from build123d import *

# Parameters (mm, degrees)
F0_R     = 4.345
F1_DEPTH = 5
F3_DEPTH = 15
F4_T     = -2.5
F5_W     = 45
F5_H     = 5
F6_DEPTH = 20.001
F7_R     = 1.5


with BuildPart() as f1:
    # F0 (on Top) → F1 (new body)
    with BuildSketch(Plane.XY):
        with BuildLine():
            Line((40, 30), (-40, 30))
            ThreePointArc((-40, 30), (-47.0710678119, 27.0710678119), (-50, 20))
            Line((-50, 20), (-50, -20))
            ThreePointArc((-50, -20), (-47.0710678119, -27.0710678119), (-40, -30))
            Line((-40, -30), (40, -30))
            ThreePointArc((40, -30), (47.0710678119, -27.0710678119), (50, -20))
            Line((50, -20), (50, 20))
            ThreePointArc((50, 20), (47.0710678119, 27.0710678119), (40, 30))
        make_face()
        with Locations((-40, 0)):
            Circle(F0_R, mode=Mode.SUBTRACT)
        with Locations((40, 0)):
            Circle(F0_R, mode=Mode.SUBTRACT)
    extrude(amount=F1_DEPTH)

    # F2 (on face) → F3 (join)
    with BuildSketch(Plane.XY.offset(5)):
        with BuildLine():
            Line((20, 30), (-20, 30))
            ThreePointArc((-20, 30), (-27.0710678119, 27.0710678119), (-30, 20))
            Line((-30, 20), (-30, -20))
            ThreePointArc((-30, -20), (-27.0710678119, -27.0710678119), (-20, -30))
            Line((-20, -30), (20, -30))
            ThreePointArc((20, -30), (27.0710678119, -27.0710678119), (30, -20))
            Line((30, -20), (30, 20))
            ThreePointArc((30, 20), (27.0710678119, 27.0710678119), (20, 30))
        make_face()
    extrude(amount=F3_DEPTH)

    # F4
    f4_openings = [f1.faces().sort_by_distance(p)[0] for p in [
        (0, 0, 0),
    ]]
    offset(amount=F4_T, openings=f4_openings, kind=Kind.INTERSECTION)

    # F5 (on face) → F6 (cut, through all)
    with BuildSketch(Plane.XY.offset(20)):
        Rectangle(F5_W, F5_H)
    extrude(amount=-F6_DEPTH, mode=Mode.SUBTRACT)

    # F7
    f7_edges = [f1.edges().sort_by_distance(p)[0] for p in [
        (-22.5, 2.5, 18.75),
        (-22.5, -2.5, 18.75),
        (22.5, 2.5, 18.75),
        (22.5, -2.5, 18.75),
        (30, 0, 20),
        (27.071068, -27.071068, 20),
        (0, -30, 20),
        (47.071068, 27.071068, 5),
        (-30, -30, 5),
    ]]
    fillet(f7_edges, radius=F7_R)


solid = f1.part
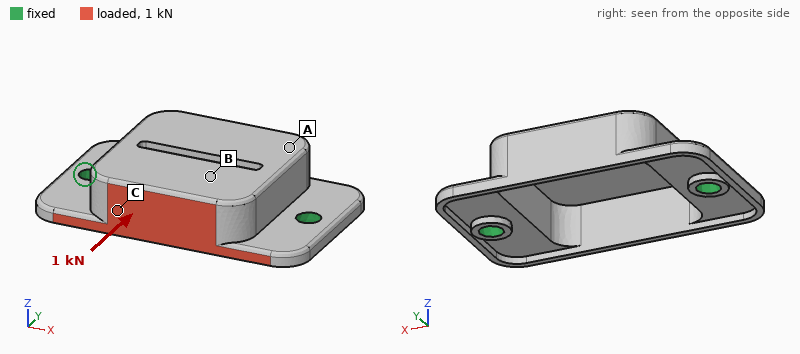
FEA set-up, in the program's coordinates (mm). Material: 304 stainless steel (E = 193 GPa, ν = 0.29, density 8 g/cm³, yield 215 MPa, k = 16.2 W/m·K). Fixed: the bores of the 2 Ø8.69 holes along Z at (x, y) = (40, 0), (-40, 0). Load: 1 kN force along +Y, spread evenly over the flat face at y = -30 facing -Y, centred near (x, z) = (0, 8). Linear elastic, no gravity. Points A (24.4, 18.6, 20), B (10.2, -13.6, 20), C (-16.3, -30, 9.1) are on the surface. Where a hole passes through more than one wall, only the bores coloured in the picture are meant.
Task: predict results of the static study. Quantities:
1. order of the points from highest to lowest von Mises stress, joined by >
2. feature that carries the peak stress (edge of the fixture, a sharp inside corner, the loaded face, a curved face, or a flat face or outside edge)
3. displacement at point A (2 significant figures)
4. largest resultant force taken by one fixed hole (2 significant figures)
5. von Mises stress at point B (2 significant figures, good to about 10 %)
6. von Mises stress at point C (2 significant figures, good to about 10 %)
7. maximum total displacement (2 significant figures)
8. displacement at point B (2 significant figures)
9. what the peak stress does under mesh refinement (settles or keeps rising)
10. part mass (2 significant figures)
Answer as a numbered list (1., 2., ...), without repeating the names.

1. C > B > A
2. a sharp inside corner
3. 11 µm
4. 540 N
5. 11 MPa
6. 56 MPa
7. 54 µm
8. 17 µm
9. keeps rising
10. 190 g
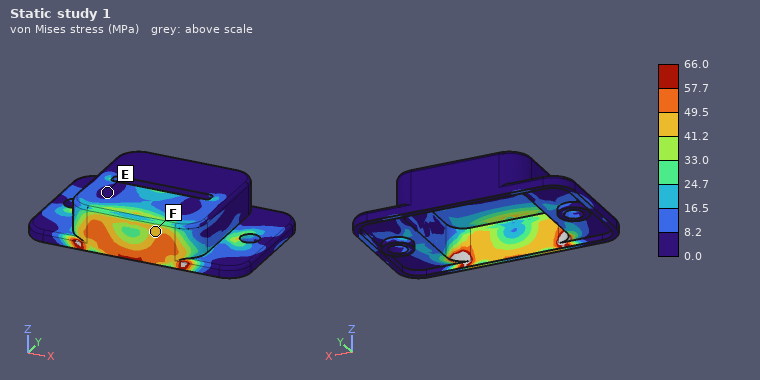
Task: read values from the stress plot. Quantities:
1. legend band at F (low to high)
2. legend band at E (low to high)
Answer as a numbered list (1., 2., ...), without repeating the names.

1. 41.2 to 49.5 MPa
2. 0.0 to 8.2 MPa
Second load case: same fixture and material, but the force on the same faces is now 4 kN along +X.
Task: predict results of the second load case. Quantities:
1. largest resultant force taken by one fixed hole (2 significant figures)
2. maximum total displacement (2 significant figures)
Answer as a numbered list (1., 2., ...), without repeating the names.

1. 2.1 kN
2. 62 µm
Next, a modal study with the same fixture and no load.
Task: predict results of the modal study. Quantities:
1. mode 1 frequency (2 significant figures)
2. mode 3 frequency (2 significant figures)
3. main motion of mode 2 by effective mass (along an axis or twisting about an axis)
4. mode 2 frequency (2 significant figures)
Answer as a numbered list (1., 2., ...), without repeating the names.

1. 1700 Hz
2. 4800 Hz
3. along Z
4. 4300 Hz
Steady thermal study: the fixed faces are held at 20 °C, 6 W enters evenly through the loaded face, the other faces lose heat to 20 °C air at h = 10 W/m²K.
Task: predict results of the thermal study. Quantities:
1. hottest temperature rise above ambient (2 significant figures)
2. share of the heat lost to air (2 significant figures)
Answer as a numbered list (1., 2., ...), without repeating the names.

1. 63 K
2. 48 %
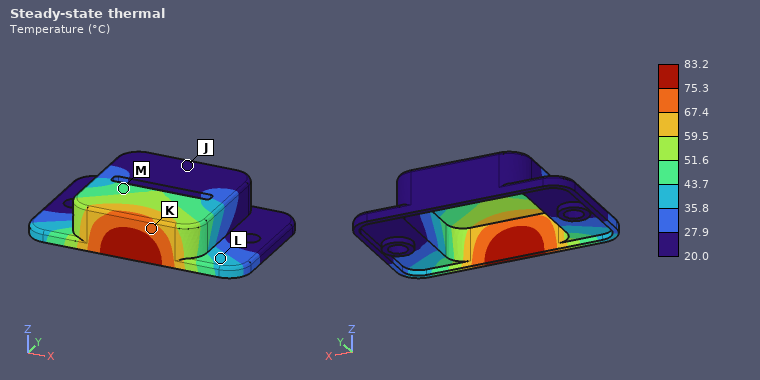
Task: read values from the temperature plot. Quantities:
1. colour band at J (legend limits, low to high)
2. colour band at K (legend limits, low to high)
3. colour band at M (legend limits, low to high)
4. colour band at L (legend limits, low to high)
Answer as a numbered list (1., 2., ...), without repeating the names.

1. 20.0 to 27.9 °C
2. 67.4 to 75.3 °C
3. 43.7 to 51.6 °C
4. 35.8 to 43.7 °C
